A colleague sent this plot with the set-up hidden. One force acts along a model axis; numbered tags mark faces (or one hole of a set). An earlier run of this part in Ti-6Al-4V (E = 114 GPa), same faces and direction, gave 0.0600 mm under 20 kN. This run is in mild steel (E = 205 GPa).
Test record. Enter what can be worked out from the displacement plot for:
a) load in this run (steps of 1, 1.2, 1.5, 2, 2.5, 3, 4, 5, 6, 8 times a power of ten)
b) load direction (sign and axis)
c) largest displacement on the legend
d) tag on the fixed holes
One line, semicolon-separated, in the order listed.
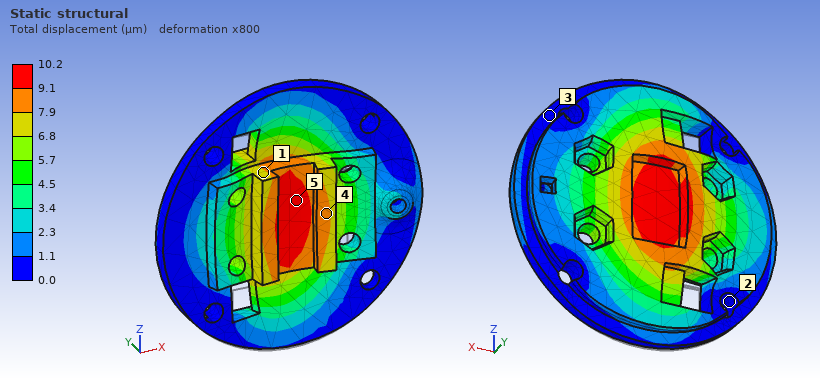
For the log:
6 kN; +Y; 10.2 µm; 2
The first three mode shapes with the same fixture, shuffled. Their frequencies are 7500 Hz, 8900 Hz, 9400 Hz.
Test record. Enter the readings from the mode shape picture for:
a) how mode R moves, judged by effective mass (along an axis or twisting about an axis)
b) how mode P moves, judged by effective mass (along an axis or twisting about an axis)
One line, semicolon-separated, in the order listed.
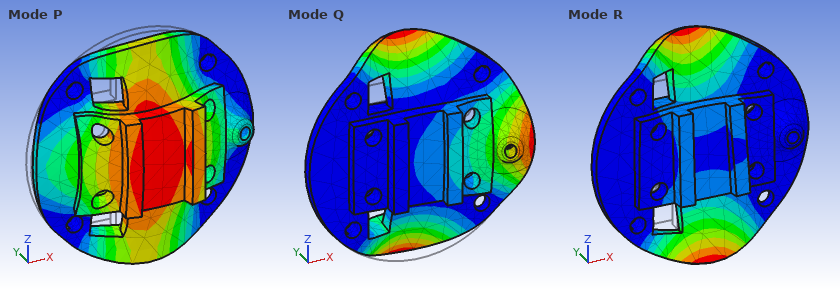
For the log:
twisting about X; along Y
